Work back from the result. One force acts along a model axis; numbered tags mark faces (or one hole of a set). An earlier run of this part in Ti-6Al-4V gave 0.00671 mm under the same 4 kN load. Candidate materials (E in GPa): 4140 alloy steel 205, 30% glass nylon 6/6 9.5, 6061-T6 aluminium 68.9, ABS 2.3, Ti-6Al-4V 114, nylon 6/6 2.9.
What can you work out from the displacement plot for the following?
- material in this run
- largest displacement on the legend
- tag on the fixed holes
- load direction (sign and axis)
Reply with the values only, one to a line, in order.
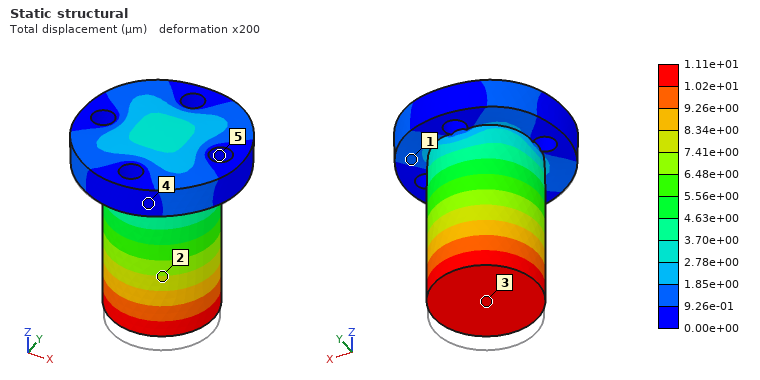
6061-T6 aluminium
1.11e+01 µm
5
+Z
